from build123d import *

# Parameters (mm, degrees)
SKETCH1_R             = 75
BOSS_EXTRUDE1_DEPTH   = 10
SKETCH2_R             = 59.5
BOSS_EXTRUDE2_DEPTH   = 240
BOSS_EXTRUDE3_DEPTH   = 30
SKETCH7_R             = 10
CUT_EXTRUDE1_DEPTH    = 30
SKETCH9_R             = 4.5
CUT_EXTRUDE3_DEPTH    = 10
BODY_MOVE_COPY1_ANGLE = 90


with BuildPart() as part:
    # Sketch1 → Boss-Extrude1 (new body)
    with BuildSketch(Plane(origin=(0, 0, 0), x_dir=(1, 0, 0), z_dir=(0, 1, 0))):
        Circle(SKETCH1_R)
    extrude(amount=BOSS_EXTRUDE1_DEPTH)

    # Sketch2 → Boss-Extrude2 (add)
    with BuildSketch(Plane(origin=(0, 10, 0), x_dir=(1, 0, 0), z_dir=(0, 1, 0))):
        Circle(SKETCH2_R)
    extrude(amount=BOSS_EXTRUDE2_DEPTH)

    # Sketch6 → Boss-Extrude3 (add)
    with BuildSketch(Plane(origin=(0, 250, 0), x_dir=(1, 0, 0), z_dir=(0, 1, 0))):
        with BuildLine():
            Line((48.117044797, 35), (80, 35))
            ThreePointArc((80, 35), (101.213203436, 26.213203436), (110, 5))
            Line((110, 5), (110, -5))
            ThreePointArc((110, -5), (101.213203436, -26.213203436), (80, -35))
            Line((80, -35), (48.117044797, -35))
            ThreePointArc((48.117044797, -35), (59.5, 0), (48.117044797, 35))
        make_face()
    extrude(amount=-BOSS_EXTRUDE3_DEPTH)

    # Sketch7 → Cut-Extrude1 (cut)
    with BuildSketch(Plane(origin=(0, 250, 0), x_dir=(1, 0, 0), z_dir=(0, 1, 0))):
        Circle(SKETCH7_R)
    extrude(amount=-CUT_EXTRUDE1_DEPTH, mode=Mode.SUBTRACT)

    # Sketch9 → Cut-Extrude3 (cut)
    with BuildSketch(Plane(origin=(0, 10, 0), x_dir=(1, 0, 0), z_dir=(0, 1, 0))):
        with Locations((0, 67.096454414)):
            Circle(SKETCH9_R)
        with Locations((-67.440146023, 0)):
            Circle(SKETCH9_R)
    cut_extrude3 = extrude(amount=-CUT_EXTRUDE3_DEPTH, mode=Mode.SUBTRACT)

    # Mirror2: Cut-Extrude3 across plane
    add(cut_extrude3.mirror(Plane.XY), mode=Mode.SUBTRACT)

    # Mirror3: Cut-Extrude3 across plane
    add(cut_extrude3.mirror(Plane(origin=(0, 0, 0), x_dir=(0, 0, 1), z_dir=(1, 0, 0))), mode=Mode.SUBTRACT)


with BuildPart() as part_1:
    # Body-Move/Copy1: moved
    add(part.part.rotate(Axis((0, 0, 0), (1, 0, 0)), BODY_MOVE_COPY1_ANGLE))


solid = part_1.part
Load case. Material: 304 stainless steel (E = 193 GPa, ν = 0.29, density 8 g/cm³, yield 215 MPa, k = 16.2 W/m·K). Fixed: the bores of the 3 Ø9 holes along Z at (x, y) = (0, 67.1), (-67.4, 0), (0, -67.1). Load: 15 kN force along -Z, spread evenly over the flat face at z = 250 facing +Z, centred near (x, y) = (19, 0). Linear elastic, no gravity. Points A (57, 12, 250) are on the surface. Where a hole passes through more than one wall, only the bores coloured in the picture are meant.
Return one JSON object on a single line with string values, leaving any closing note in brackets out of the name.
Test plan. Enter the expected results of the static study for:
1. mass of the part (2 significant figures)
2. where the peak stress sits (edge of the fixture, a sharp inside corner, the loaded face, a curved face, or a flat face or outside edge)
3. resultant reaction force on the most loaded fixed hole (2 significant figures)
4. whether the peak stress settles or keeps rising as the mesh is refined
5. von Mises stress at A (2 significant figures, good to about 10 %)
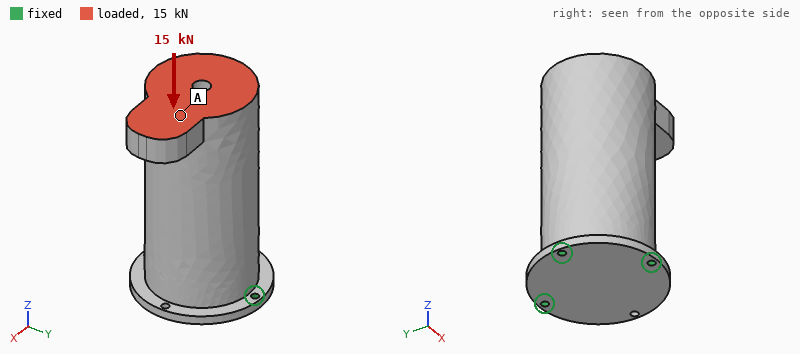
{"mass of the part": "23 kg", "where the peak stress sits": "edge of the fixture", "resultant reaction force on the most loaded fixed hole": "10 kN", "whether the peak stress settles or keeps rising as the mesh is refined": "keeps rising", "von Mises stress at A": "6.4 MPa"}
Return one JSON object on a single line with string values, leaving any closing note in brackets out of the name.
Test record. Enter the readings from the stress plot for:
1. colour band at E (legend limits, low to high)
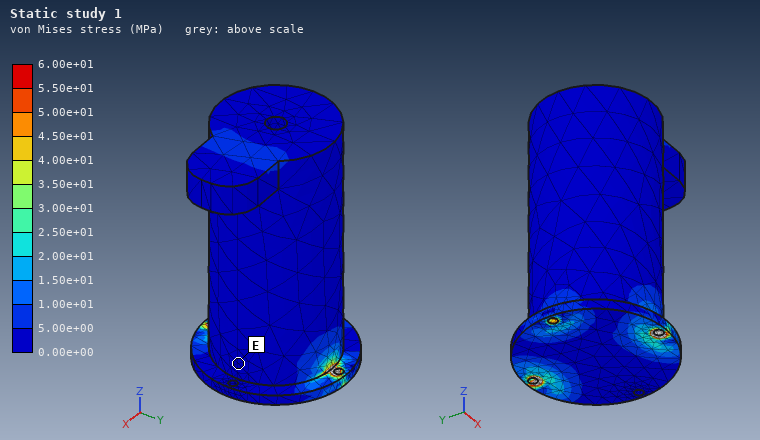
{"colour band at E": "0.00e+00 to 5.00e+00 MPa"}
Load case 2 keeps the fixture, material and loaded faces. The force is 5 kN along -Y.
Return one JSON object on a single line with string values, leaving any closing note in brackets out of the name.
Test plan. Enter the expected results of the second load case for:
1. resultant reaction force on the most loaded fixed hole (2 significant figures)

{"resultant reaction force on the most loaded fixed hole": "10 kN"}
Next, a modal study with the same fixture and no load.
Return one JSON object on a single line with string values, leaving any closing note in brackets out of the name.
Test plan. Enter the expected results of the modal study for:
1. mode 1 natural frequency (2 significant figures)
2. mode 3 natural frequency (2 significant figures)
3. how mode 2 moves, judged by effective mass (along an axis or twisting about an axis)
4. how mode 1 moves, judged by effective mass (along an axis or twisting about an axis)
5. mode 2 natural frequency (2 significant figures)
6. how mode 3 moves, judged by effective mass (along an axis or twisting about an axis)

{"mode 1 natural frequency": "340 Hz", "mode 3 natural frequency": "1700 Hz", "how mode 2 moves, judged by effective mass": "along Y", "how mode 1 moves, judged by effective mass": "along X", "mode 2 natural frequency": "570 Hz", "how mode 3 moves, judged by effective mass": "along Z"}
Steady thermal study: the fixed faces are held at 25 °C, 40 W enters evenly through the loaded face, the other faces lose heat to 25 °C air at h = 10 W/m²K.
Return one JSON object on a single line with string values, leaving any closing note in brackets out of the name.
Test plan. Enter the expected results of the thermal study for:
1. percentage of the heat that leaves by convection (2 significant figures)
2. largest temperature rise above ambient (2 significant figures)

{"percentage of the heat that leaves by convection": "70 %", "largest temperature rise above ambient": "49 K"}
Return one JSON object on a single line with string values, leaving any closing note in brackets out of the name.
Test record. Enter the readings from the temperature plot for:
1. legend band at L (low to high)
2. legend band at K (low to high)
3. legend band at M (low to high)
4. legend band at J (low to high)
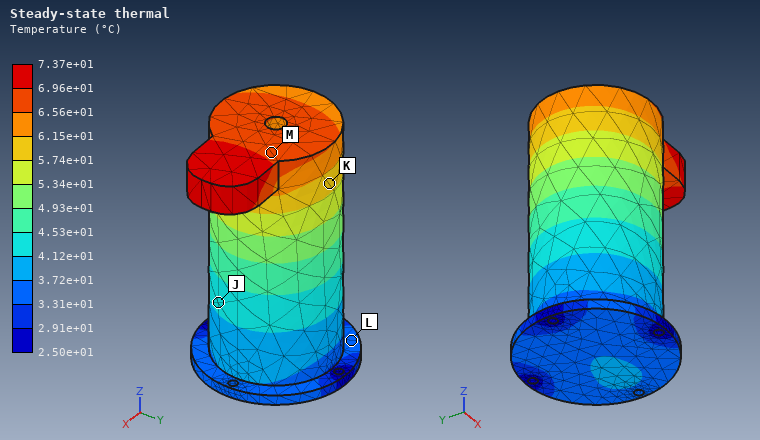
{"legend band at L": "3.31e+01 to 3.72e+01 °C", "legend band at K": "5.74e+01 to 6.15e+01 °C", "legend band at M": "6.56e+01 to 6.96e+01 °C", "legend band at J": "4.12e+01 to 4.53e+01 °C"}
